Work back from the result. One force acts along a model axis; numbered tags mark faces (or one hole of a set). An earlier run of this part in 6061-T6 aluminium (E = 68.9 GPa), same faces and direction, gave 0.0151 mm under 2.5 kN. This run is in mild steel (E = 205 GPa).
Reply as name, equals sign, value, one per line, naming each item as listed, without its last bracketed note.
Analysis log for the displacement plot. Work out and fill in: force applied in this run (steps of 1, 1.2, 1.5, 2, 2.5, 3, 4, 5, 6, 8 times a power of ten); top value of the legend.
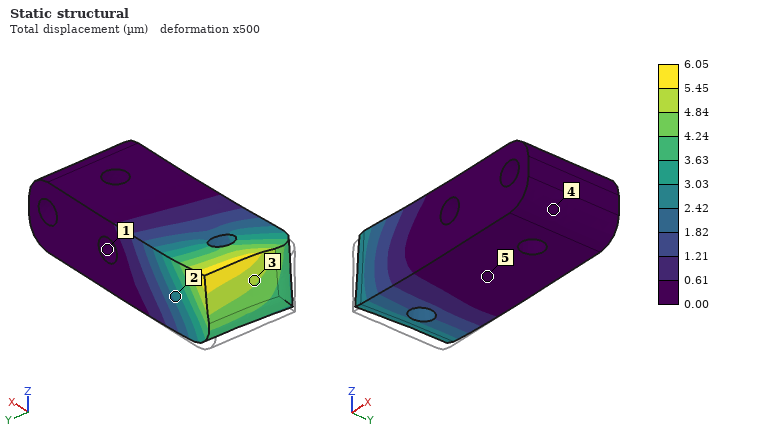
force applied in this run = 3 kN
top value of the legend = 6.05 µm
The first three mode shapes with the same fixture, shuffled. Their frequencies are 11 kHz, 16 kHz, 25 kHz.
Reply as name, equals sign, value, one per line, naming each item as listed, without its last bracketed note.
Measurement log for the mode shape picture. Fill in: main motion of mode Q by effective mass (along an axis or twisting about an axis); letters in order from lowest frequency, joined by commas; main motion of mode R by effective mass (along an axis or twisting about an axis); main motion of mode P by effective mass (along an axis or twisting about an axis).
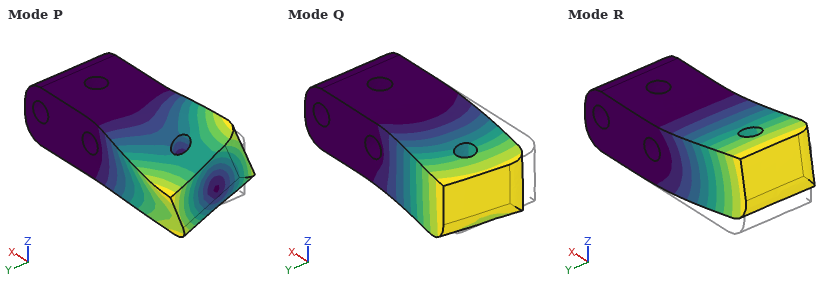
main motion of mode Q by effective mass = along Y
letters in order from lowest frequency, joined by commas = R, Q, P
main motion of mode R by effective mass = along Z
main motion of mode P by effective mass = twisting about X
